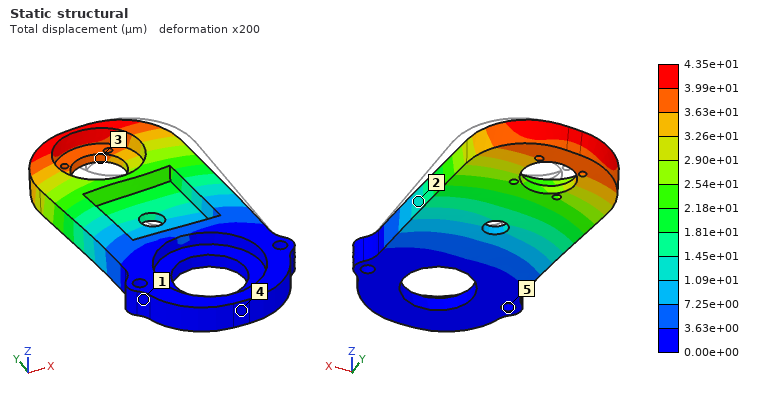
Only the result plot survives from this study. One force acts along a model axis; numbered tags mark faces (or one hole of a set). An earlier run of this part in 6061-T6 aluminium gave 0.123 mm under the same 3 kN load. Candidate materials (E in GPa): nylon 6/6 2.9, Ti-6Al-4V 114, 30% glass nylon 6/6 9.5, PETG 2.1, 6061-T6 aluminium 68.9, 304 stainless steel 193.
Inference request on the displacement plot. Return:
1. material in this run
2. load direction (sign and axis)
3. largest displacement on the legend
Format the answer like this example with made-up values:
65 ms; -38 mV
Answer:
304 stainless steel; -X; 4.35e+01 µm
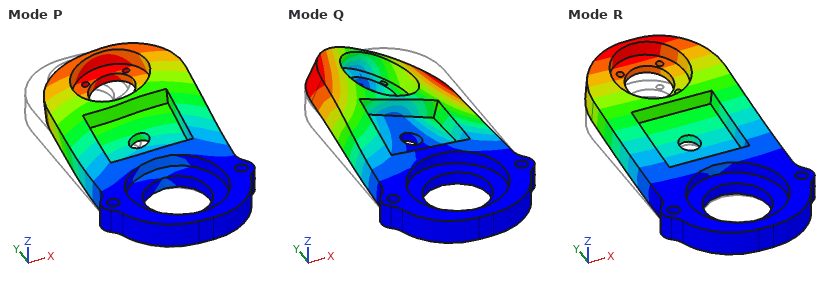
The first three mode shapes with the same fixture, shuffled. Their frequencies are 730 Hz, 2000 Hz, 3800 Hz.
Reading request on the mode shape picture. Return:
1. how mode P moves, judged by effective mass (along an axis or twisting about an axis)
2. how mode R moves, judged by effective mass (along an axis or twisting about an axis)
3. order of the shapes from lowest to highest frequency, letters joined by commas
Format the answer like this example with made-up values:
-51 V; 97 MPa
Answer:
along X; along Z; R, Q, P
